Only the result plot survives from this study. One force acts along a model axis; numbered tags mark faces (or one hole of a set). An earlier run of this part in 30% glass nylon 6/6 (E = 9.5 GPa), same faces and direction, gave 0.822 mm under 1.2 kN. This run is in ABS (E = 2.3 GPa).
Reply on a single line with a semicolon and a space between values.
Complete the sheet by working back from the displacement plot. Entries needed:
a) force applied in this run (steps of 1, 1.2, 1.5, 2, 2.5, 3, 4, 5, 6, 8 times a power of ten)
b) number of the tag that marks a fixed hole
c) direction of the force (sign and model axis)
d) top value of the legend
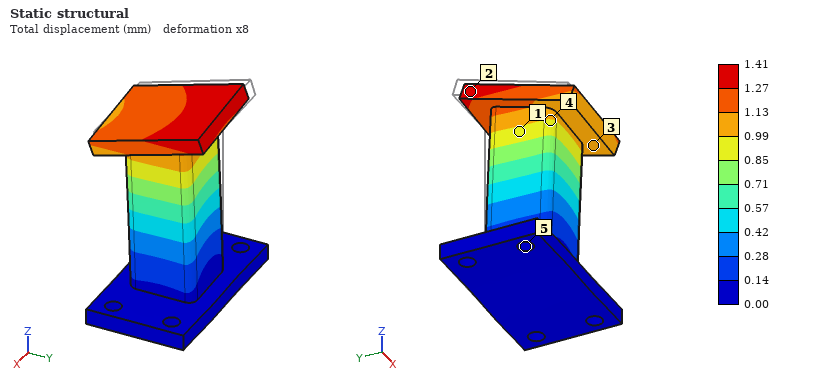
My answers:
500 N; 5; +X; 1.41 mm
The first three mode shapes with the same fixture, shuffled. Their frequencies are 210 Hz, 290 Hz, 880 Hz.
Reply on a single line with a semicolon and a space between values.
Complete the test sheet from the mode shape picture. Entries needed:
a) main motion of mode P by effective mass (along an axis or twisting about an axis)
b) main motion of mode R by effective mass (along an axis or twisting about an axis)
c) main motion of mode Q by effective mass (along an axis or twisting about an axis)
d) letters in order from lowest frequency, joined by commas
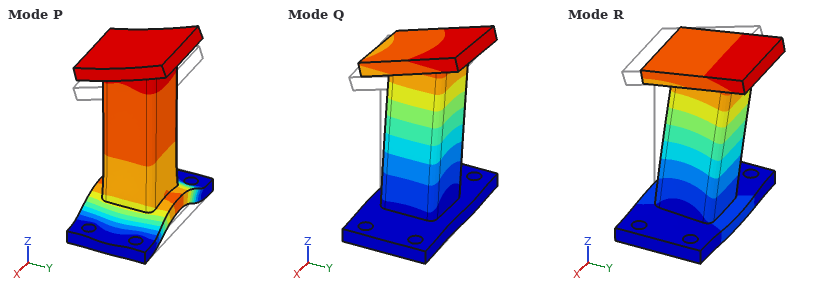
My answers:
along Z; along Y; along X; R, Q, P
